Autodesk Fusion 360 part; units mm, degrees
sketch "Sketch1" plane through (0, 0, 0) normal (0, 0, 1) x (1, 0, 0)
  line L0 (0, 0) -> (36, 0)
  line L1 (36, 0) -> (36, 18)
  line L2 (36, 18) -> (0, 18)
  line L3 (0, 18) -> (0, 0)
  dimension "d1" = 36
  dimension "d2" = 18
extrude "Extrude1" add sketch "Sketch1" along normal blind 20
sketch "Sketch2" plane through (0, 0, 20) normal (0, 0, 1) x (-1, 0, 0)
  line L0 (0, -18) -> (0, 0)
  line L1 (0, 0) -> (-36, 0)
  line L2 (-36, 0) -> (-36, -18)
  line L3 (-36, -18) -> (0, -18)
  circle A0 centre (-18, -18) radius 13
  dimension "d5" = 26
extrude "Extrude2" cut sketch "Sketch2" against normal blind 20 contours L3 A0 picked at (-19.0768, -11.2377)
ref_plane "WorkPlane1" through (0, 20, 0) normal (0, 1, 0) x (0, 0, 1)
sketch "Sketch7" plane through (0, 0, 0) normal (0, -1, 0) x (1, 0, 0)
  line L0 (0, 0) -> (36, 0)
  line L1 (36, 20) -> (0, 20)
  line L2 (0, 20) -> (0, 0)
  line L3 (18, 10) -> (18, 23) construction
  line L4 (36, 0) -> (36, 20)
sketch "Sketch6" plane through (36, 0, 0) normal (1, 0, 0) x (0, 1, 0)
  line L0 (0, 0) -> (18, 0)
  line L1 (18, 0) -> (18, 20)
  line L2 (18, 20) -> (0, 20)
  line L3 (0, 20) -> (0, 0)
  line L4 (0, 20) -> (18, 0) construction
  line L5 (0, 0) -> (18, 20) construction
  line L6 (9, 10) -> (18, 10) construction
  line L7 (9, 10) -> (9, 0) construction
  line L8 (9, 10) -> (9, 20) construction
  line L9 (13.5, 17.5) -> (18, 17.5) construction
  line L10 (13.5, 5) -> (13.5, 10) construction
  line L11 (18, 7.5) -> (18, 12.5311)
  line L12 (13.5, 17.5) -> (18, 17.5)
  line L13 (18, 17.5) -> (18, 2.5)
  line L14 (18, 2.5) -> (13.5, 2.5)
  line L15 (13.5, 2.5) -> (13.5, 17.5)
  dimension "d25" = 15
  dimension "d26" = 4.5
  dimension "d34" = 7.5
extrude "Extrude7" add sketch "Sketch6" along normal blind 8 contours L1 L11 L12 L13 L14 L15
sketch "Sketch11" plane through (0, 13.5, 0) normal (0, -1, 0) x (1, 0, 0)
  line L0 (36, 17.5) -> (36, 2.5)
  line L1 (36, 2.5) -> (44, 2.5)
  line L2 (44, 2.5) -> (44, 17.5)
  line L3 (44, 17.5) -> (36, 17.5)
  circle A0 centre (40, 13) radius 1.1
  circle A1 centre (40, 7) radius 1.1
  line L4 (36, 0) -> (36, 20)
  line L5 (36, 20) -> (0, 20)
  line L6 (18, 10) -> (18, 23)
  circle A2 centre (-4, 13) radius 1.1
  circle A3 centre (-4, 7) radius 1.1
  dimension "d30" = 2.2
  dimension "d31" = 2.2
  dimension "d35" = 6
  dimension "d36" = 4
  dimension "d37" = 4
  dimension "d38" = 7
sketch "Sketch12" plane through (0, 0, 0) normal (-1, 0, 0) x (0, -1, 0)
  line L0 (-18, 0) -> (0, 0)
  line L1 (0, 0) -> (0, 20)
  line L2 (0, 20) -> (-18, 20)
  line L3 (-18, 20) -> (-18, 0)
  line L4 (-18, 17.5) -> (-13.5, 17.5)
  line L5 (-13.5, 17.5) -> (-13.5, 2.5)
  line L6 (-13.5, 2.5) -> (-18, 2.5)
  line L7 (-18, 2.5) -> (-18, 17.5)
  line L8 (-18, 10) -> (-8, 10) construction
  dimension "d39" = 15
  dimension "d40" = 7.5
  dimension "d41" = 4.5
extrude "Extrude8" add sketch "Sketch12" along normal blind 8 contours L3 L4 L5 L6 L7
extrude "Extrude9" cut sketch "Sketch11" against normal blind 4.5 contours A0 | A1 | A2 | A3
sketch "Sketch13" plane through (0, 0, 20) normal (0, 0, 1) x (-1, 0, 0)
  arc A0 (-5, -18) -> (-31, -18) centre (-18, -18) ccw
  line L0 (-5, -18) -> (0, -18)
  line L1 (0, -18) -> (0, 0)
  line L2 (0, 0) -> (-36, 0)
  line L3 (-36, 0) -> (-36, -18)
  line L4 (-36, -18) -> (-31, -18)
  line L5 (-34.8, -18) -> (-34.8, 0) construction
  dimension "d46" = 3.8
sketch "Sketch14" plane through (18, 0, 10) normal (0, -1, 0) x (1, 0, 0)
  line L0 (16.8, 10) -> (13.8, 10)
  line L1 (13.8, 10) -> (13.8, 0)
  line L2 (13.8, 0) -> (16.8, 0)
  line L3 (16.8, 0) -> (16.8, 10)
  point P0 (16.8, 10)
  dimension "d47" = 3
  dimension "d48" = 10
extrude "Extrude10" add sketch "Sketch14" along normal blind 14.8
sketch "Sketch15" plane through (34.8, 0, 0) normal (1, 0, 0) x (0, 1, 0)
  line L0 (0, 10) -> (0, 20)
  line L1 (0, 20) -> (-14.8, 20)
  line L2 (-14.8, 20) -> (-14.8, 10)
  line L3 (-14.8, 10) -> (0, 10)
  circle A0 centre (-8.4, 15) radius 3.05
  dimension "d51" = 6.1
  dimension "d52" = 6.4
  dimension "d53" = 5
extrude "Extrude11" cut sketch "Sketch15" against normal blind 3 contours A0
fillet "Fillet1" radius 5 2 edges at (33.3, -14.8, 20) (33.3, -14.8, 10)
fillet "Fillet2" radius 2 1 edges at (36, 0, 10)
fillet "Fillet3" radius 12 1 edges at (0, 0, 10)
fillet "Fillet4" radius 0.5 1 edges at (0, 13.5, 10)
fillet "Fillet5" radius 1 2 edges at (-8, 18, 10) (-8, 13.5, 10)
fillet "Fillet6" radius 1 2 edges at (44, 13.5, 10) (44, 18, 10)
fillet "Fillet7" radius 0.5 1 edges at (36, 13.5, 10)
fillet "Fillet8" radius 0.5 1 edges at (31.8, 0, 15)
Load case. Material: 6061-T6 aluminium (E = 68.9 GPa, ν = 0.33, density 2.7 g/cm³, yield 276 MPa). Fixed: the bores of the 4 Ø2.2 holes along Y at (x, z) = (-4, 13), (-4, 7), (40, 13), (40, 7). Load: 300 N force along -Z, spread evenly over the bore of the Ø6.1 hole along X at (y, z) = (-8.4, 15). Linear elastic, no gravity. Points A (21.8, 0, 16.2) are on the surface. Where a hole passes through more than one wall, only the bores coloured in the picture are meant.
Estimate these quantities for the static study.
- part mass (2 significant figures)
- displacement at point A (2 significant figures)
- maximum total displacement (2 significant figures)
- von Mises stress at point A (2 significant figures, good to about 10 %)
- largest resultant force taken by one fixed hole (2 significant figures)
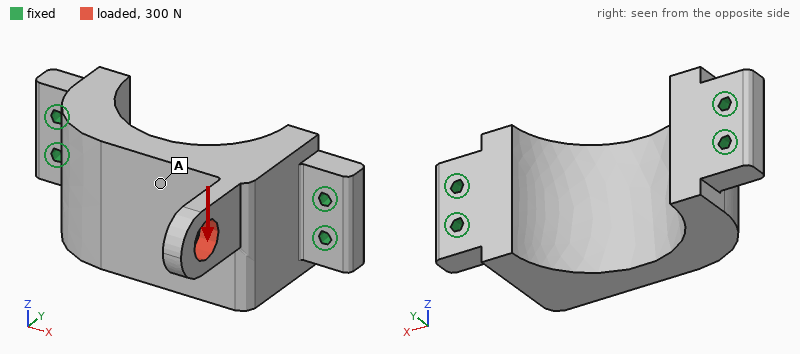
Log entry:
23 g
21 µm
75 µm
12 MPa
450 N
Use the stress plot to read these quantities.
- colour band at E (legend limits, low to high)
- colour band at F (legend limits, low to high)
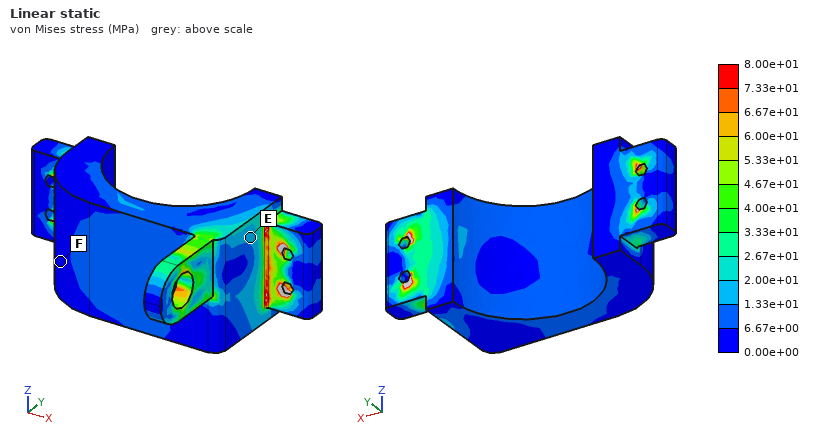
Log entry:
1.33e+01 to 2.00e+01 MPa
0.00e+00 to 6.67e+00 MPa
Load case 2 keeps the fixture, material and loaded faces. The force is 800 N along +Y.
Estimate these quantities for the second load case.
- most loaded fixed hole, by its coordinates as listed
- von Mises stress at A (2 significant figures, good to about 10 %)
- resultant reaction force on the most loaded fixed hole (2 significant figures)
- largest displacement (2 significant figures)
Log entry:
(40, 13)
7.5 MPa
610 N
34 µm
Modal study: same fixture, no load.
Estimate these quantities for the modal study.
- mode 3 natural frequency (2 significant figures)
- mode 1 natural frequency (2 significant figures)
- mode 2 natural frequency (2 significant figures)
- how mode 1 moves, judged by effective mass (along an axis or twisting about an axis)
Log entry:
16 kHz
7000 Hz
11 kHz
along Z
